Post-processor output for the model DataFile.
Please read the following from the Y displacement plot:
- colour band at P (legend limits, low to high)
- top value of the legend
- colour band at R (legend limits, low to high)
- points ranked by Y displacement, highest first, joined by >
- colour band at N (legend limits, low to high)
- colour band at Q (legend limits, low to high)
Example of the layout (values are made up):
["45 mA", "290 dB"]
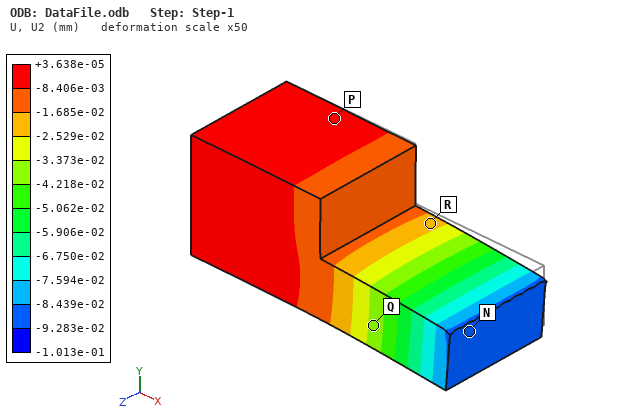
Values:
["-8.406e-03 to +3.638e-05 mm", "+3.638e-05 mm", "-2.529e-02 to -1.685e-02 mm", "P > R > Q > N", "-9.283e-02 to -8.439e-02 mm", "-4.218e-02 to -3.373e-02 mm"]
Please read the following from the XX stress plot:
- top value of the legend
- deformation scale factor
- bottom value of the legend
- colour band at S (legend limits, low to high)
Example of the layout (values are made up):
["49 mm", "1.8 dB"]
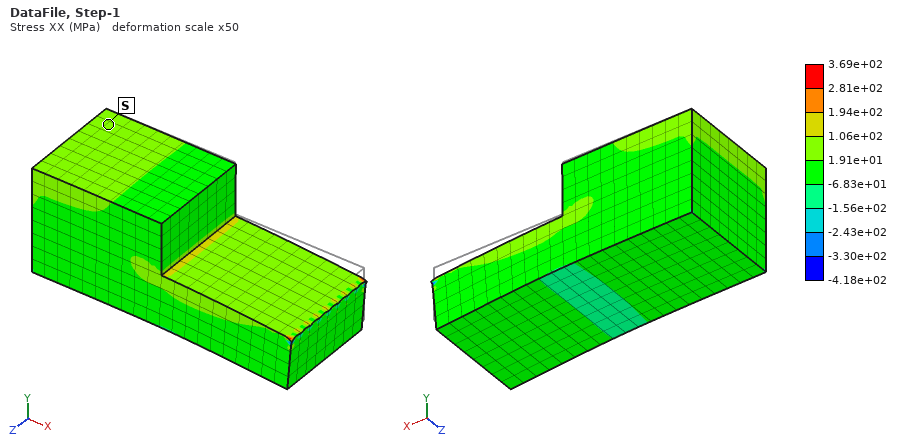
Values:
["3.69e+02 MPa", "50", "-4.18e+02 MPa", "1.91e+01 to 1.06e+02 MPa"]
